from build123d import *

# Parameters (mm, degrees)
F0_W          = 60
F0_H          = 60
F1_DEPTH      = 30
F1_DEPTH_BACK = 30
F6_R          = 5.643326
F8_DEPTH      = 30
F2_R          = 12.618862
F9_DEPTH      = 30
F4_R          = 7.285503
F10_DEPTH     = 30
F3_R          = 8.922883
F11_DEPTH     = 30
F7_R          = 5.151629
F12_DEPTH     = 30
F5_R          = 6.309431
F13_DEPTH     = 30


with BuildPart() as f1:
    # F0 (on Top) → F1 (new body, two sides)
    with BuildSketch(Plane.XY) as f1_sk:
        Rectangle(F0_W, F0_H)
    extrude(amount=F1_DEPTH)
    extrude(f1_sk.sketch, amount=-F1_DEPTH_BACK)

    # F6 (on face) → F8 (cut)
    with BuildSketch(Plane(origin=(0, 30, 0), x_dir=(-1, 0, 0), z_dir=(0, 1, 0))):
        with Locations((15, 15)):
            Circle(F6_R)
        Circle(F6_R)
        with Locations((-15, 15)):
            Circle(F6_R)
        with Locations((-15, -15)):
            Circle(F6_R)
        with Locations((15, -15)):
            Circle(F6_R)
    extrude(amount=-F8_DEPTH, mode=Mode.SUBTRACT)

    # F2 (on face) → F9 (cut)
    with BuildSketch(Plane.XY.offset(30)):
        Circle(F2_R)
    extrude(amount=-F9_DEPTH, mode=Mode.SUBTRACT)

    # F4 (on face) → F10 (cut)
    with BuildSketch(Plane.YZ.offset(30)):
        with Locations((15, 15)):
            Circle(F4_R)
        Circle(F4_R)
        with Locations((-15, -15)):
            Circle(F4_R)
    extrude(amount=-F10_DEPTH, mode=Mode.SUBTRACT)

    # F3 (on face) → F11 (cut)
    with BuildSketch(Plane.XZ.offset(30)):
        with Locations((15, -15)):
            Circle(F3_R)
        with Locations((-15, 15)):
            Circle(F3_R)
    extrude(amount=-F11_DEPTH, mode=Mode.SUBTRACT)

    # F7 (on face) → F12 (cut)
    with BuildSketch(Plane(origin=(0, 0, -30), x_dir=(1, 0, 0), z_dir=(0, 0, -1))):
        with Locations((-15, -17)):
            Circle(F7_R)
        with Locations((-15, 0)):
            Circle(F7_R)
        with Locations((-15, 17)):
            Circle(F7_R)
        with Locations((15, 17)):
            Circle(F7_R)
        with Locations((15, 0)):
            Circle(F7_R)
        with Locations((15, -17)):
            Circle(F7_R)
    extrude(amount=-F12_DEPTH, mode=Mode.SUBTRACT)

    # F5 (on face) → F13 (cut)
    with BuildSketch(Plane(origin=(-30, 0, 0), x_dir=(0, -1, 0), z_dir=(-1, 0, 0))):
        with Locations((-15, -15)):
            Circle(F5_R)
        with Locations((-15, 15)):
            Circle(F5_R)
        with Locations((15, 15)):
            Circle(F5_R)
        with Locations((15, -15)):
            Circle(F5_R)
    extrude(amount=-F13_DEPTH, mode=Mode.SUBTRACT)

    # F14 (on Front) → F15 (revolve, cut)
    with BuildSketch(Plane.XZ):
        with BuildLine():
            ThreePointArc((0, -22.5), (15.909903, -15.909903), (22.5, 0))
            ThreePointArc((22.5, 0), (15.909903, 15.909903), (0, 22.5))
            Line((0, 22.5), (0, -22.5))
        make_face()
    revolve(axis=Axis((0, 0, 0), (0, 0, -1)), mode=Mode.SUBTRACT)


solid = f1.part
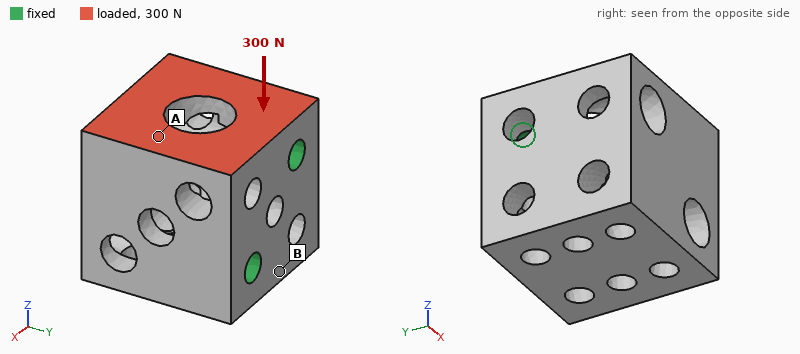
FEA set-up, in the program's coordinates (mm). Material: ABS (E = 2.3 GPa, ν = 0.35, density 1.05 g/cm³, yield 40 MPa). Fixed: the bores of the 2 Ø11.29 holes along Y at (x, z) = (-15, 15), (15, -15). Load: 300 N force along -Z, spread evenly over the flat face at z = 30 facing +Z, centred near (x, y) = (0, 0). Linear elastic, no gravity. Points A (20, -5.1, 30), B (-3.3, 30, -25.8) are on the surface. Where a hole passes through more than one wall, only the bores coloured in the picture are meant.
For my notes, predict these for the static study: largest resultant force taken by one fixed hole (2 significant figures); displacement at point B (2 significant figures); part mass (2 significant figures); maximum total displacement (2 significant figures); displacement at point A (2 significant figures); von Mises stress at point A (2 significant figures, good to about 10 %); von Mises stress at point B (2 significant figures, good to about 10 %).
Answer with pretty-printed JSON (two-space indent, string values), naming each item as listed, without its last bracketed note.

{
  "largest resultant force taken by one fixed hole": "170 N",
  "displacement at point B": "9.2 µm",
  "part mass": "130 g",
  "maximum total displacement": "50 µm",
  "displacement at point A": "37 µm",
  "von Mises stress at point A": "0.17 MPa",
  "von Mises stress at point B": "0.35 MPa"
}
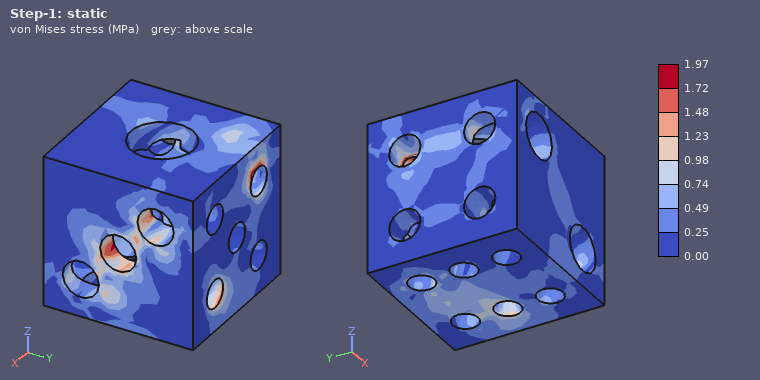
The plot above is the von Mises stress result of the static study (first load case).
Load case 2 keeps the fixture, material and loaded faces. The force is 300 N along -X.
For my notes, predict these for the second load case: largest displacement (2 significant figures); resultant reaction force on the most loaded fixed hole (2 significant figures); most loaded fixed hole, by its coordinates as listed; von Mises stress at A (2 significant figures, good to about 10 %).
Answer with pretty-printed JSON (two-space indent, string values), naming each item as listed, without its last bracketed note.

{
  "largest displacement": "76 µm",
  "resultant reaction force on the most loaded fixed hole": "300 N",
  "most loaded fixed hole, by its coordinates as listed": "(-15, 15)",
  "von Mises stress at A": "0.51 MPa"
}
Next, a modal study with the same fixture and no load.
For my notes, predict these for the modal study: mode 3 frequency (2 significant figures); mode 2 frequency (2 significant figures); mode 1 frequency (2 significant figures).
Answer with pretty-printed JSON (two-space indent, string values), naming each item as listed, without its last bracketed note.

{
  "mode 3 frequency": "2600 Hz",
  "mode 2 frequency": "1800 Hz",
  "mode 1 frequency": "1100 Hz"
}
